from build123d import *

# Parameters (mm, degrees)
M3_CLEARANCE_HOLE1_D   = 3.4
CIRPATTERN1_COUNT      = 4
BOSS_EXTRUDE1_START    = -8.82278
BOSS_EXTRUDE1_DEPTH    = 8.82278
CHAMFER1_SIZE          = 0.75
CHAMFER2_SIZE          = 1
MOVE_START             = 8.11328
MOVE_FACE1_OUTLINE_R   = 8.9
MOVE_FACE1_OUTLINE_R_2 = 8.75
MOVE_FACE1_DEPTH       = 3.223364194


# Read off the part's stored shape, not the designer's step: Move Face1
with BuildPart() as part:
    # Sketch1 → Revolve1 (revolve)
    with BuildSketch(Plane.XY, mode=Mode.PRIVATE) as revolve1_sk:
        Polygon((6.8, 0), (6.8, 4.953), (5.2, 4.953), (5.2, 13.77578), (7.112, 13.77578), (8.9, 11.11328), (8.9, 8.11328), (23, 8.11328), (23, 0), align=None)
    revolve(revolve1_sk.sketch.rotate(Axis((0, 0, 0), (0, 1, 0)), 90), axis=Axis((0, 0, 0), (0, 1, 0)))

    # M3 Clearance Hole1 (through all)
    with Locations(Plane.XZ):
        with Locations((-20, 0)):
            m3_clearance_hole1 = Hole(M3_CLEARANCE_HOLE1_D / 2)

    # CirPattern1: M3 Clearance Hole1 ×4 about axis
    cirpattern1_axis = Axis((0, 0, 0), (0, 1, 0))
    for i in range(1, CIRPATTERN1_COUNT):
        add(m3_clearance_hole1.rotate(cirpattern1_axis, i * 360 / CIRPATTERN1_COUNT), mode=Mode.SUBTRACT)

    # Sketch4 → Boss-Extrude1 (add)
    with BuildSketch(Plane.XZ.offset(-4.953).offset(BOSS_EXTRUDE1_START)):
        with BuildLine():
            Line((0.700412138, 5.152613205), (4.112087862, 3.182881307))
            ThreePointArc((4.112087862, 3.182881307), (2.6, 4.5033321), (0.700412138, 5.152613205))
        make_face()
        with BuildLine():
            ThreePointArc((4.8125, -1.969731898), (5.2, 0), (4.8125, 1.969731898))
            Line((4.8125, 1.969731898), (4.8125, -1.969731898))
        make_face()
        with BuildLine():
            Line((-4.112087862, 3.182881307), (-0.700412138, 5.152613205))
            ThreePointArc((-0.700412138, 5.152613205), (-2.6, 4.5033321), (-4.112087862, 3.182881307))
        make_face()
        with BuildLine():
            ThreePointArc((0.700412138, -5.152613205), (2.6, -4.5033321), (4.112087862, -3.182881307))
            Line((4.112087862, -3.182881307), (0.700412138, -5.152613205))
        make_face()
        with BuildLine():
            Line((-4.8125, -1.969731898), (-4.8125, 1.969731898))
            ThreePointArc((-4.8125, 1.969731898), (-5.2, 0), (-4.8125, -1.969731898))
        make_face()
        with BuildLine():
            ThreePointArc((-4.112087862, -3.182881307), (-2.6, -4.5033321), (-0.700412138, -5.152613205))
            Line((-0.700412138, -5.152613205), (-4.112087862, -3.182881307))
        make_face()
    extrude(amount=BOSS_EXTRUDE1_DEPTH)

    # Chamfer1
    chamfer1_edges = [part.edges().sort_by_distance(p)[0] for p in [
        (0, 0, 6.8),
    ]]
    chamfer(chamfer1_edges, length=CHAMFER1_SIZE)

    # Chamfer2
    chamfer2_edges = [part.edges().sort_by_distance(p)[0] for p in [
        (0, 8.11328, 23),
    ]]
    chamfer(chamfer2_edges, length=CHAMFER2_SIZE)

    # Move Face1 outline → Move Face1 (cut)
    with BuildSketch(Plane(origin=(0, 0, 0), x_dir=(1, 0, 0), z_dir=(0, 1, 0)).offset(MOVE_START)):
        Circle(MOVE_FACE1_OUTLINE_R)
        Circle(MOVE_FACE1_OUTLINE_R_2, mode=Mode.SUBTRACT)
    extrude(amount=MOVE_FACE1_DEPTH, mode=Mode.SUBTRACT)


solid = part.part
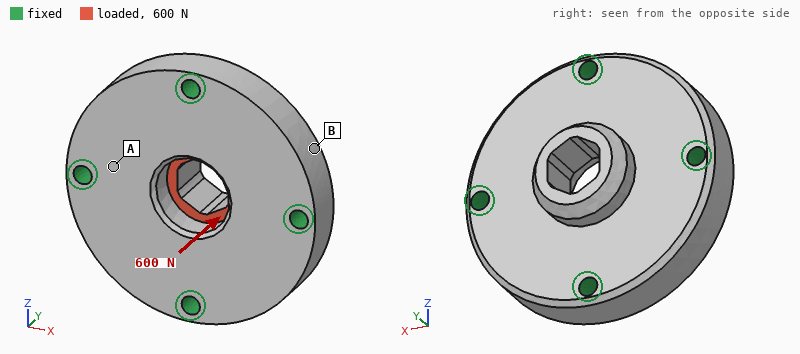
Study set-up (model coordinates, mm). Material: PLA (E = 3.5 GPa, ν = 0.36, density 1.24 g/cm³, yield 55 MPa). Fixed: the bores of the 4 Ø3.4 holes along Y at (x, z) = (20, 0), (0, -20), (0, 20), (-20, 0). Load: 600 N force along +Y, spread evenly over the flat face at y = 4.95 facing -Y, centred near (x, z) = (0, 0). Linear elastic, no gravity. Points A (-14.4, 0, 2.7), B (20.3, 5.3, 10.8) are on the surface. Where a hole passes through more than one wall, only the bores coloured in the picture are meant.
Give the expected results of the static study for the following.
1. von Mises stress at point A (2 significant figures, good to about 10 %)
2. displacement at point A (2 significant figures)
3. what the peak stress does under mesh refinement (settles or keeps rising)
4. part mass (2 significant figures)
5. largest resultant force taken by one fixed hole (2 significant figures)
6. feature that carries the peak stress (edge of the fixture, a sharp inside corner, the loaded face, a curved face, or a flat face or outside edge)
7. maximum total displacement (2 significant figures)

3.1 MPa
17 µm
keeps rising
16 g
160 N
edge of the fixture
51 µm
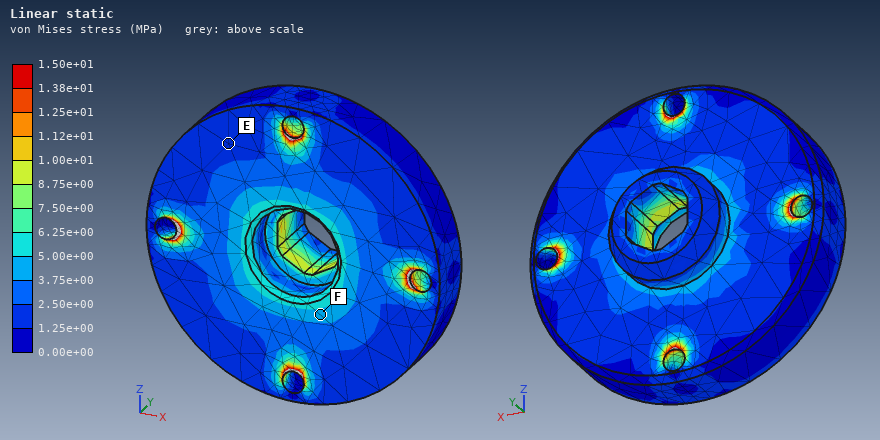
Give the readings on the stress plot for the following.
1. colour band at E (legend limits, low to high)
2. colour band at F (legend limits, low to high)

1.25e+00 to 2.50e+00 MPa
3.75e+00 to 5.00e+00 MPa
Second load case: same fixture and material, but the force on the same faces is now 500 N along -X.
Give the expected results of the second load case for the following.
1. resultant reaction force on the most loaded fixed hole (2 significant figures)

160 N
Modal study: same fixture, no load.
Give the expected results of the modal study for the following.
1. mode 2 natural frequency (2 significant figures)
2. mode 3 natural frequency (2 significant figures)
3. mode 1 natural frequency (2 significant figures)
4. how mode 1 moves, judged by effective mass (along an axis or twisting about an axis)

11 kHz
11 kHz
9200 Hz
along Y
